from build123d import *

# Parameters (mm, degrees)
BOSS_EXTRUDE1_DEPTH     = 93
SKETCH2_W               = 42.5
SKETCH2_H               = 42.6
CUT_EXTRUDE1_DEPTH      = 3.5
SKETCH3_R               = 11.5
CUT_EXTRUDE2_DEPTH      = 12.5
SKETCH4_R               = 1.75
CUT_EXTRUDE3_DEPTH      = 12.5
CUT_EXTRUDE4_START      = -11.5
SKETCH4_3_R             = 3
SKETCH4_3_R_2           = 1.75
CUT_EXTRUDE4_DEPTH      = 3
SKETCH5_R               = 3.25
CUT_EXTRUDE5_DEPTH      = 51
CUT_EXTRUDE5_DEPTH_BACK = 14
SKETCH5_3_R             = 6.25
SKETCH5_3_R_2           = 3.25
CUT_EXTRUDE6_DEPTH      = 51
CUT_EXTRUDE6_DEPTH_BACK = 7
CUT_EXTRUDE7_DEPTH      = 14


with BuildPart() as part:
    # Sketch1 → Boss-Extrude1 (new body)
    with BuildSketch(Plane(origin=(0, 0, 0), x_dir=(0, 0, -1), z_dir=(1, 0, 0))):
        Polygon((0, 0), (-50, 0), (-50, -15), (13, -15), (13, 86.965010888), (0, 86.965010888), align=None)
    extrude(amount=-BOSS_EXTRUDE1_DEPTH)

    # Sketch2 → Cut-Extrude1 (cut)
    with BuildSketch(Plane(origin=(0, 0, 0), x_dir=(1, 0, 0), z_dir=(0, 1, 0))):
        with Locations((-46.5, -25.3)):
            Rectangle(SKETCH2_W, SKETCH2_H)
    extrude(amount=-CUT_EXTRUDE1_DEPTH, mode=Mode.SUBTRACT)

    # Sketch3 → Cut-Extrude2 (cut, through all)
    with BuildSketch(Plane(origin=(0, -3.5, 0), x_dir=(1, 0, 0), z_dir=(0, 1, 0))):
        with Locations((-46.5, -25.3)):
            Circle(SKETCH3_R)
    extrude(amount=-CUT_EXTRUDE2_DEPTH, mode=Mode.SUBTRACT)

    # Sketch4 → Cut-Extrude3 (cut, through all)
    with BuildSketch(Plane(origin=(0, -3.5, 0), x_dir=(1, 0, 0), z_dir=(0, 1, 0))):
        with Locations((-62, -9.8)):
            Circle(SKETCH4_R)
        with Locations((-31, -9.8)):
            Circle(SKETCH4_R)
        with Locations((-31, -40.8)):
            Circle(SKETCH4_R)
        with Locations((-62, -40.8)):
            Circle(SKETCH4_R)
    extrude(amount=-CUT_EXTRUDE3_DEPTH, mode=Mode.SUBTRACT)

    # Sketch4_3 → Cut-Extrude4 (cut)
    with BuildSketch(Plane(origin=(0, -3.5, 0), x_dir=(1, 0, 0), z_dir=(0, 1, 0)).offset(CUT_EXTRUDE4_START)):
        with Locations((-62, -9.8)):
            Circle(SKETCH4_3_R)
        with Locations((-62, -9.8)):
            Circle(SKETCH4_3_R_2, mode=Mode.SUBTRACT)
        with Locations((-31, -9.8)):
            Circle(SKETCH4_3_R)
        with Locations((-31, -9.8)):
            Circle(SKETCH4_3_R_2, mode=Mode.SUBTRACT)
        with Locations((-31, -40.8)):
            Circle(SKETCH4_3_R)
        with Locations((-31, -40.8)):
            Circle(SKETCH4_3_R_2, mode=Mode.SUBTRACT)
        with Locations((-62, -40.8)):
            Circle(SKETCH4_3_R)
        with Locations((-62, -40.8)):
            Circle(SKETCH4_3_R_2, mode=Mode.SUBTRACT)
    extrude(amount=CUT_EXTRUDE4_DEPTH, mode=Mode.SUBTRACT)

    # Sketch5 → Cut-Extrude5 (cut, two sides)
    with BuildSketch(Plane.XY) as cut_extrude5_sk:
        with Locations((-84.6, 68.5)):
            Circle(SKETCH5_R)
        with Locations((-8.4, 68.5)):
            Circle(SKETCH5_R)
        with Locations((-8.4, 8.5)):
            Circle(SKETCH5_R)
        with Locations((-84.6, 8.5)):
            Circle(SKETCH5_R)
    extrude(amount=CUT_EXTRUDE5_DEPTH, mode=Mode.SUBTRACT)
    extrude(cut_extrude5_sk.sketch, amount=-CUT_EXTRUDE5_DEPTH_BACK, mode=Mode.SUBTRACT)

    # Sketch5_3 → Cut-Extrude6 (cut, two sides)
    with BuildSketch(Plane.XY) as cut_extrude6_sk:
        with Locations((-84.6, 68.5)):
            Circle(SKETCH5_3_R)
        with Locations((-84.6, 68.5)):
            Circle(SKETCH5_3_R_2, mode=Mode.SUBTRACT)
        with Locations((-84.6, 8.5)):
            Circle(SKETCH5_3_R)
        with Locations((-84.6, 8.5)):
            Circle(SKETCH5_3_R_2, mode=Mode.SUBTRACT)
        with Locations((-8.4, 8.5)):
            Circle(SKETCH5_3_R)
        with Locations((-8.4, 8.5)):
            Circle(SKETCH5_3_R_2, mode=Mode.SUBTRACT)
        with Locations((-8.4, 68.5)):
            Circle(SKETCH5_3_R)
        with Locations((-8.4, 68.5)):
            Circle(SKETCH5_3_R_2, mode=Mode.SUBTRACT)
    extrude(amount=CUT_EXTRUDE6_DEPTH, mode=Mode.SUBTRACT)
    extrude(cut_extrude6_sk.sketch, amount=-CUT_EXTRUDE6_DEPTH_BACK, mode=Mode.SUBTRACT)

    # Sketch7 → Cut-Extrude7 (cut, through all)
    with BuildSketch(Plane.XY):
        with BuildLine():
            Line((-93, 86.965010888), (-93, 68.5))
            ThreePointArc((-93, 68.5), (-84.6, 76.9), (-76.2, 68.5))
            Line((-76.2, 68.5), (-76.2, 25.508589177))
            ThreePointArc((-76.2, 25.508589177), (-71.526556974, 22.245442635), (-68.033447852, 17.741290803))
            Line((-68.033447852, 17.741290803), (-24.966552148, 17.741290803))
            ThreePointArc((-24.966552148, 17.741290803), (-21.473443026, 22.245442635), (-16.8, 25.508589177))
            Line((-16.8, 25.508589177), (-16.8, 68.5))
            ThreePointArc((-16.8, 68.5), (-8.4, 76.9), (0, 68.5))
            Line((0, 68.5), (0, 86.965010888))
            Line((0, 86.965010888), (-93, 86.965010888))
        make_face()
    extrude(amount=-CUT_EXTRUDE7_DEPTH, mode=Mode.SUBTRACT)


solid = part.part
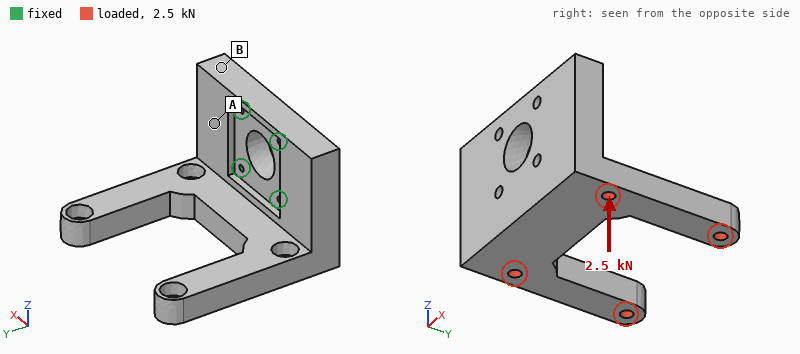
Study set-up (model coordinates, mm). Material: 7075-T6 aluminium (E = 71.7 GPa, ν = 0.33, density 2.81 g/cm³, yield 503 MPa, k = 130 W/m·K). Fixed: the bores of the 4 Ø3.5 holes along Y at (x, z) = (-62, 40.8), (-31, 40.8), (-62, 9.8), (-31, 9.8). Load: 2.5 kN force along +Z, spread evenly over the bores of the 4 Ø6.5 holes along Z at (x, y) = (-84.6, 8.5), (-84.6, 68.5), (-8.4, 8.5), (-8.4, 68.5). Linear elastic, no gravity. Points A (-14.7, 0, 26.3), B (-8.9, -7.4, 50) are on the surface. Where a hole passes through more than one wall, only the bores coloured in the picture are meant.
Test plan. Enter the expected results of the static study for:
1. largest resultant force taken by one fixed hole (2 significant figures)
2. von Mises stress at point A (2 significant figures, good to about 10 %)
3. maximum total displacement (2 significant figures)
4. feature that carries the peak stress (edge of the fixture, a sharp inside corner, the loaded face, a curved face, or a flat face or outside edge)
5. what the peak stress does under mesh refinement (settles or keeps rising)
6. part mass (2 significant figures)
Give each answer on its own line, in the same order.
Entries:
1.7 kN
21 MPa
0.56 mm
edge of the fixture
keeps rising
340 g
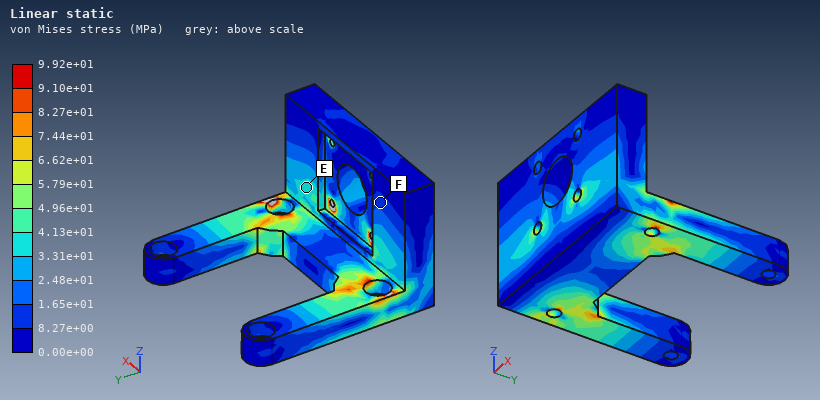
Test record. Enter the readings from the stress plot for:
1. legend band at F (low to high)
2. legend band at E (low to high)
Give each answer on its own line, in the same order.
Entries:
8.27e+00 to 1.65e+01 MPa
3.31e+01 to 4.13e+01 MPa
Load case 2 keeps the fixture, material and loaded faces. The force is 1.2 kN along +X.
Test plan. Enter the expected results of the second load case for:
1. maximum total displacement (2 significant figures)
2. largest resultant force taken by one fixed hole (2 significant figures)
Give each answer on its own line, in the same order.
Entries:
0.11 mm
1.6 kN
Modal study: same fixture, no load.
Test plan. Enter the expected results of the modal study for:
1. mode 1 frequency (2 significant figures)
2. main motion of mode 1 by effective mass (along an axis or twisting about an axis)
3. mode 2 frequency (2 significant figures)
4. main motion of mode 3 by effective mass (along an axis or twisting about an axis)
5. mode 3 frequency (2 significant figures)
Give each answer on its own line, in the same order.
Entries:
1600 Hz
along Z
1800 Hz
along X
2500 Hz
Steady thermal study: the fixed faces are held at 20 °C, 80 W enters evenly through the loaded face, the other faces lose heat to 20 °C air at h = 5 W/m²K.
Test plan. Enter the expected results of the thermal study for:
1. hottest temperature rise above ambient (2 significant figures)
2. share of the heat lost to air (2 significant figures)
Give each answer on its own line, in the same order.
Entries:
72 K
3.7 %
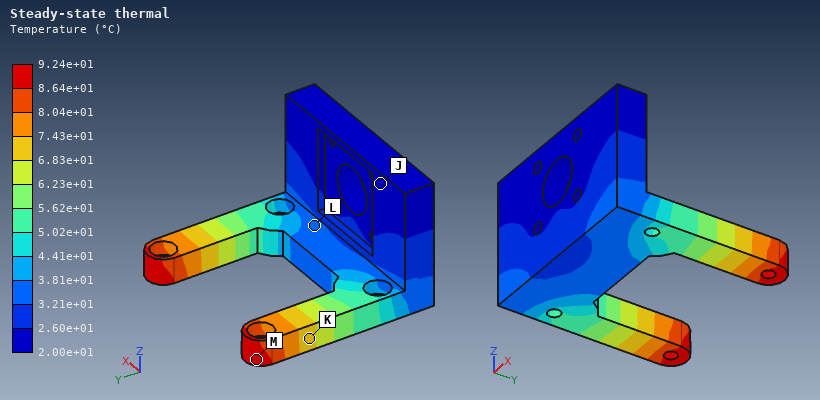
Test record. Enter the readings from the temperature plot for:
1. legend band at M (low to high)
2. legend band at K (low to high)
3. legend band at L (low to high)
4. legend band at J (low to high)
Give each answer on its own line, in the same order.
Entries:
8.64e+01 to 9.24e+01 °C
6.83e+01 to 7.43e+01 °C
3.21e+01 to 3.81e+01 °C
2.00e+01 to 2.60e+01 °C
